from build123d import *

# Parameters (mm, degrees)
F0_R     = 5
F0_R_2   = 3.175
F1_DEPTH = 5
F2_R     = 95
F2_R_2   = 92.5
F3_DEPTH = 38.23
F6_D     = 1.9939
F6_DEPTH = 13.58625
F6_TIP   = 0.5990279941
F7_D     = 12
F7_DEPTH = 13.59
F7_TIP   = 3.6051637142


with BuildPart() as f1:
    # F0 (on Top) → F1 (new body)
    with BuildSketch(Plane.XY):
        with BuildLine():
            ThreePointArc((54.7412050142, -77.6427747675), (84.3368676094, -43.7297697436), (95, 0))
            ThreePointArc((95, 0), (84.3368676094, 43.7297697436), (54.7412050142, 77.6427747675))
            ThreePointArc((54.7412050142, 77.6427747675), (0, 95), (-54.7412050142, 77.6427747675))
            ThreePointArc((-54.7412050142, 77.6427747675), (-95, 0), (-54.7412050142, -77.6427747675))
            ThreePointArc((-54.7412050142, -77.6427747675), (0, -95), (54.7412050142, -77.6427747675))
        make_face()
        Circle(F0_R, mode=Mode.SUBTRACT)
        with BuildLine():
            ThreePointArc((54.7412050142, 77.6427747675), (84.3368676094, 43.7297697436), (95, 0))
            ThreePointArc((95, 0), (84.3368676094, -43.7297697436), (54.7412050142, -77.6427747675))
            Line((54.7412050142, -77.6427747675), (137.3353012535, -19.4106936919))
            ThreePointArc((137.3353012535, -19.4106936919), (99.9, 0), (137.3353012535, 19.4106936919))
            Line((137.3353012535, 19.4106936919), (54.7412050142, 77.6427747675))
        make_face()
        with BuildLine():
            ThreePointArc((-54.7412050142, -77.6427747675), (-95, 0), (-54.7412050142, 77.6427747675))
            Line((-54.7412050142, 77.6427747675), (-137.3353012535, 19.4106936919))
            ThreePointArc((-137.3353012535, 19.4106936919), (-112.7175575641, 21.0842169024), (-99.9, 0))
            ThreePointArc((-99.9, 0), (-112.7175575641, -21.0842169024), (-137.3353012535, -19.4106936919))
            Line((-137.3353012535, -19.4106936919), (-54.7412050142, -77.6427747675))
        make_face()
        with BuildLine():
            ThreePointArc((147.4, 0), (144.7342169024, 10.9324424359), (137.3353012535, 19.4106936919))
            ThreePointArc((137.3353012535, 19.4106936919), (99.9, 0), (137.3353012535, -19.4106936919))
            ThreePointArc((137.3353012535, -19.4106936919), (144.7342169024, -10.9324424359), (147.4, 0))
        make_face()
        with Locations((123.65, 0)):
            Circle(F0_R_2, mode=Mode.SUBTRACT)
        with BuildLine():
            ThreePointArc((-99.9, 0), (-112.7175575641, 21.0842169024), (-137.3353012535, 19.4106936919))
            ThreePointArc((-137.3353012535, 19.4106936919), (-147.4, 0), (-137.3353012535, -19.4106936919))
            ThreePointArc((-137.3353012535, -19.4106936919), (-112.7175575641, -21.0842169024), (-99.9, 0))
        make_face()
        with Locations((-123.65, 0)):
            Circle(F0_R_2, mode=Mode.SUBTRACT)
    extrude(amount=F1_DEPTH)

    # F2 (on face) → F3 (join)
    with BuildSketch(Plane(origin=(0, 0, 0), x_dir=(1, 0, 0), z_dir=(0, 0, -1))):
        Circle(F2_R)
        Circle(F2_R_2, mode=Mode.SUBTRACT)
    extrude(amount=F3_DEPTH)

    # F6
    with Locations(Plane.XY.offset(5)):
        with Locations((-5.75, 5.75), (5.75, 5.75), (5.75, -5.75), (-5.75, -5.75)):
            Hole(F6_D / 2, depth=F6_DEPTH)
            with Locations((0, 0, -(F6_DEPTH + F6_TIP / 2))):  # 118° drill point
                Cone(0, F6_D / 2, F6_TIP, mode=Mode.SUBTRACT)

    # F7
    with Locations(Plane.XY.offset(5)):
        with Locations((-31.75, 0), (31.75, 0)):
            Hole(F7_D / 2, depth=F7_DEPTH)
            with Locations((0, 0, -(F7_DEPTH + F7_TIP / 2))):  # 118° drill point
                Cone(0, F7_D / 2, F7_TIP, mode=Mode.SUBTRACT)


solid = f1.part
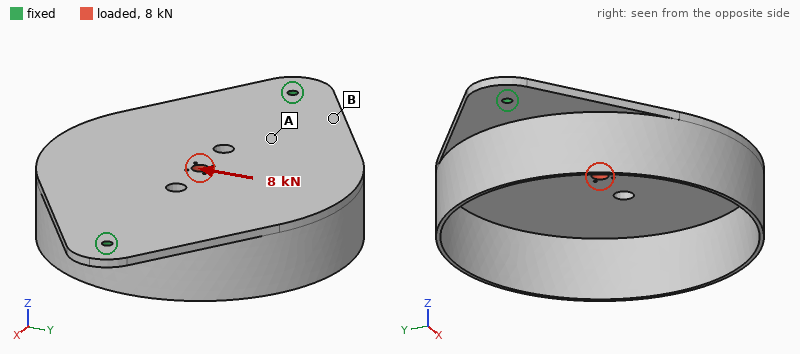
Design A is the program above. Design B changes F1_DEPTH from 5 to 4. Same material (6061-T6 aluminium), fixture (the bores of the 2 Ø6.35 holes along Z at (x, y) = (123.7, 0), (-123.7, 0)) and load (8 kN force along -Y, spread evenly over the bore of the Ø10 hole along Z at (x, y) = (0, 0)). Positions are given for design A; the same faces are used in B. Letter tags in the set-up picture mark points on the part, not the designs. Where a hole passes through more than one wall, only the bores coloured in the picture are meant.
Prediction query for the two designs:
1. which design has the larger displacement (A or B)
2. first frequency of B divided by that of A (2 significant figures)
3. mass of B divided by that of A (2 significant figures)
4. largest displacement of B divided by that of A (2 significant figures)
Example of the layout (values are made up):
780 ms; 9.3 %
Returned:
B; 0.80; 0.85; 1.2
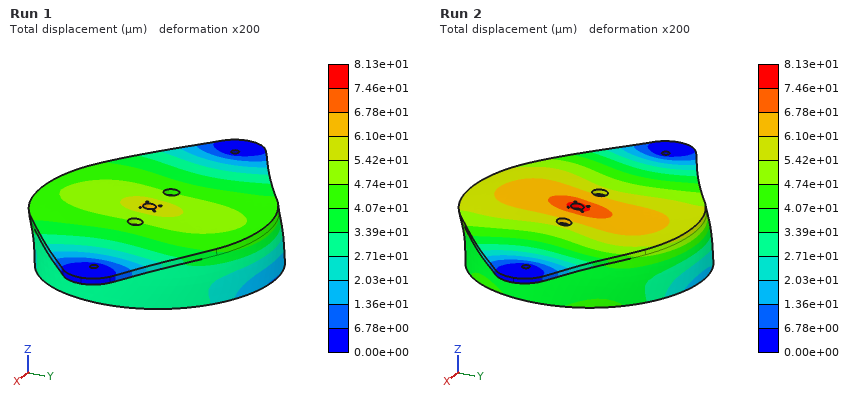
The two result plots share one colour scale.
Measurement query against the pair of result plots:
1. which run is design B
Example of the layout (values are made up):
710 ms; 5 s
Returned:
Run 2
